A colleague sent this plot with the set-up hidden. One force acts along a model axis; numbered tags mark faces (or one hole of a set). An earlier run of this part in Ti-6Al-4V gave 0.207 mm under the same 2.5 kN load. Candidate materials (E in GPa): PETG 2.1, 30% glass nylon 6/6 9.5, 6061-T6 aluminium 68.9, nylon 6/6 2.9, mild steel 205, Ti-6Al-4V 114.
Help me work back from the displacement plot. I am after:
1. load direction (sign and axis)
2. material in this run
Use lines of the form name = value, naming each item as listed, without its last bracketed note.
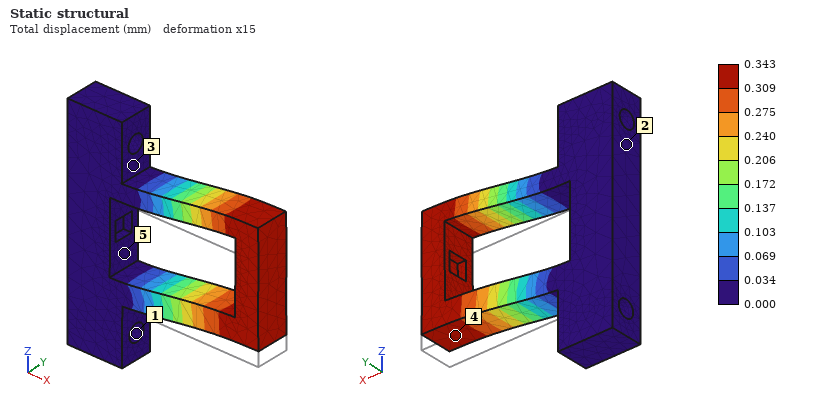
load direction = +Z
material in this run = 6061-T6 aluminium
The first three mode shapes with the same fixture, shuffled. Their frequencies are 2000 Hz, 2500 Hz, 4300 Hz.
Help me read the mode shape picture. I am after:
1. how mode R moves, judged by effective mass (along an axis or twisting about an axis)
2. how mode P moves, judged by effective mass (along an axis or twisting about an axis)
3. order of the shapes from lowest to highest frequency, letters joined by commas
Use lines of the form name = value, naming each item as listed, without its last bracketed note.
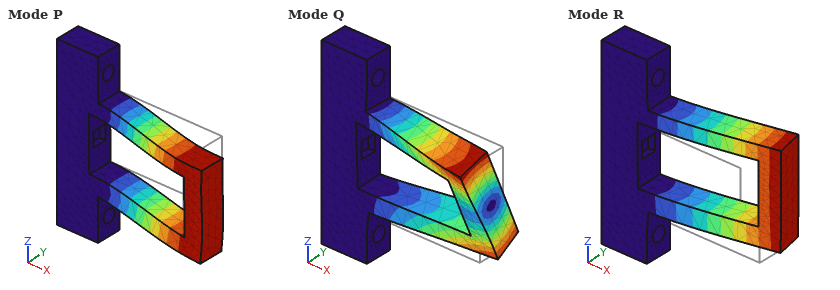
how mode R moves, judged by effective mass = along Y
how mode P moves, judged by effective mass = along Z
order of the shapes from lowest to highest frequency, letters joined by commas = R, P, Q
